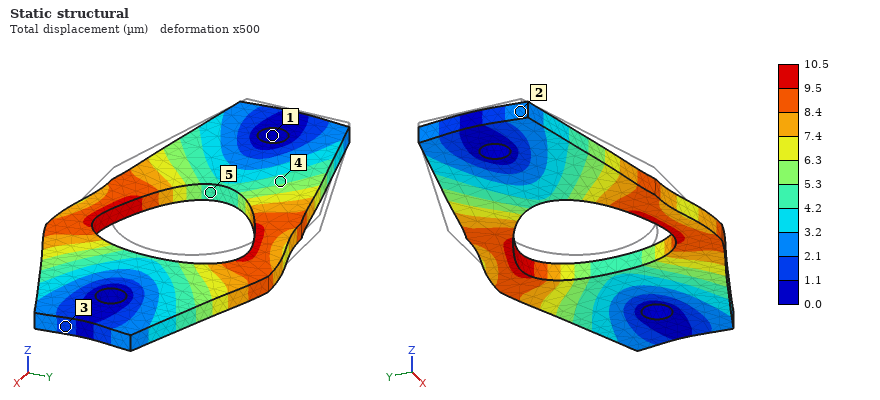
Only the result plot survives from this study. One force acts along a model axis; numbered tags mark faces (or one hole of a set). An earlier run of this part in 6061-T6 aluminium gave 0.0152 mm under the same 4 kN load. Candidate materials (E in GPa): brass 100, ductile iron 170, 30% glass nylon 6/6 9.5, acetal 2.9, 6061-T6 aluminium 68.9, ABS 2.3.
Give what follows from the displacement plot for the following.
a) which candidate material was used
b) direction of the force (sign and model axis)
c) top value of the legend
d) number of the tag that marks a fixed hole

brass
+X
10.5 µm
1
